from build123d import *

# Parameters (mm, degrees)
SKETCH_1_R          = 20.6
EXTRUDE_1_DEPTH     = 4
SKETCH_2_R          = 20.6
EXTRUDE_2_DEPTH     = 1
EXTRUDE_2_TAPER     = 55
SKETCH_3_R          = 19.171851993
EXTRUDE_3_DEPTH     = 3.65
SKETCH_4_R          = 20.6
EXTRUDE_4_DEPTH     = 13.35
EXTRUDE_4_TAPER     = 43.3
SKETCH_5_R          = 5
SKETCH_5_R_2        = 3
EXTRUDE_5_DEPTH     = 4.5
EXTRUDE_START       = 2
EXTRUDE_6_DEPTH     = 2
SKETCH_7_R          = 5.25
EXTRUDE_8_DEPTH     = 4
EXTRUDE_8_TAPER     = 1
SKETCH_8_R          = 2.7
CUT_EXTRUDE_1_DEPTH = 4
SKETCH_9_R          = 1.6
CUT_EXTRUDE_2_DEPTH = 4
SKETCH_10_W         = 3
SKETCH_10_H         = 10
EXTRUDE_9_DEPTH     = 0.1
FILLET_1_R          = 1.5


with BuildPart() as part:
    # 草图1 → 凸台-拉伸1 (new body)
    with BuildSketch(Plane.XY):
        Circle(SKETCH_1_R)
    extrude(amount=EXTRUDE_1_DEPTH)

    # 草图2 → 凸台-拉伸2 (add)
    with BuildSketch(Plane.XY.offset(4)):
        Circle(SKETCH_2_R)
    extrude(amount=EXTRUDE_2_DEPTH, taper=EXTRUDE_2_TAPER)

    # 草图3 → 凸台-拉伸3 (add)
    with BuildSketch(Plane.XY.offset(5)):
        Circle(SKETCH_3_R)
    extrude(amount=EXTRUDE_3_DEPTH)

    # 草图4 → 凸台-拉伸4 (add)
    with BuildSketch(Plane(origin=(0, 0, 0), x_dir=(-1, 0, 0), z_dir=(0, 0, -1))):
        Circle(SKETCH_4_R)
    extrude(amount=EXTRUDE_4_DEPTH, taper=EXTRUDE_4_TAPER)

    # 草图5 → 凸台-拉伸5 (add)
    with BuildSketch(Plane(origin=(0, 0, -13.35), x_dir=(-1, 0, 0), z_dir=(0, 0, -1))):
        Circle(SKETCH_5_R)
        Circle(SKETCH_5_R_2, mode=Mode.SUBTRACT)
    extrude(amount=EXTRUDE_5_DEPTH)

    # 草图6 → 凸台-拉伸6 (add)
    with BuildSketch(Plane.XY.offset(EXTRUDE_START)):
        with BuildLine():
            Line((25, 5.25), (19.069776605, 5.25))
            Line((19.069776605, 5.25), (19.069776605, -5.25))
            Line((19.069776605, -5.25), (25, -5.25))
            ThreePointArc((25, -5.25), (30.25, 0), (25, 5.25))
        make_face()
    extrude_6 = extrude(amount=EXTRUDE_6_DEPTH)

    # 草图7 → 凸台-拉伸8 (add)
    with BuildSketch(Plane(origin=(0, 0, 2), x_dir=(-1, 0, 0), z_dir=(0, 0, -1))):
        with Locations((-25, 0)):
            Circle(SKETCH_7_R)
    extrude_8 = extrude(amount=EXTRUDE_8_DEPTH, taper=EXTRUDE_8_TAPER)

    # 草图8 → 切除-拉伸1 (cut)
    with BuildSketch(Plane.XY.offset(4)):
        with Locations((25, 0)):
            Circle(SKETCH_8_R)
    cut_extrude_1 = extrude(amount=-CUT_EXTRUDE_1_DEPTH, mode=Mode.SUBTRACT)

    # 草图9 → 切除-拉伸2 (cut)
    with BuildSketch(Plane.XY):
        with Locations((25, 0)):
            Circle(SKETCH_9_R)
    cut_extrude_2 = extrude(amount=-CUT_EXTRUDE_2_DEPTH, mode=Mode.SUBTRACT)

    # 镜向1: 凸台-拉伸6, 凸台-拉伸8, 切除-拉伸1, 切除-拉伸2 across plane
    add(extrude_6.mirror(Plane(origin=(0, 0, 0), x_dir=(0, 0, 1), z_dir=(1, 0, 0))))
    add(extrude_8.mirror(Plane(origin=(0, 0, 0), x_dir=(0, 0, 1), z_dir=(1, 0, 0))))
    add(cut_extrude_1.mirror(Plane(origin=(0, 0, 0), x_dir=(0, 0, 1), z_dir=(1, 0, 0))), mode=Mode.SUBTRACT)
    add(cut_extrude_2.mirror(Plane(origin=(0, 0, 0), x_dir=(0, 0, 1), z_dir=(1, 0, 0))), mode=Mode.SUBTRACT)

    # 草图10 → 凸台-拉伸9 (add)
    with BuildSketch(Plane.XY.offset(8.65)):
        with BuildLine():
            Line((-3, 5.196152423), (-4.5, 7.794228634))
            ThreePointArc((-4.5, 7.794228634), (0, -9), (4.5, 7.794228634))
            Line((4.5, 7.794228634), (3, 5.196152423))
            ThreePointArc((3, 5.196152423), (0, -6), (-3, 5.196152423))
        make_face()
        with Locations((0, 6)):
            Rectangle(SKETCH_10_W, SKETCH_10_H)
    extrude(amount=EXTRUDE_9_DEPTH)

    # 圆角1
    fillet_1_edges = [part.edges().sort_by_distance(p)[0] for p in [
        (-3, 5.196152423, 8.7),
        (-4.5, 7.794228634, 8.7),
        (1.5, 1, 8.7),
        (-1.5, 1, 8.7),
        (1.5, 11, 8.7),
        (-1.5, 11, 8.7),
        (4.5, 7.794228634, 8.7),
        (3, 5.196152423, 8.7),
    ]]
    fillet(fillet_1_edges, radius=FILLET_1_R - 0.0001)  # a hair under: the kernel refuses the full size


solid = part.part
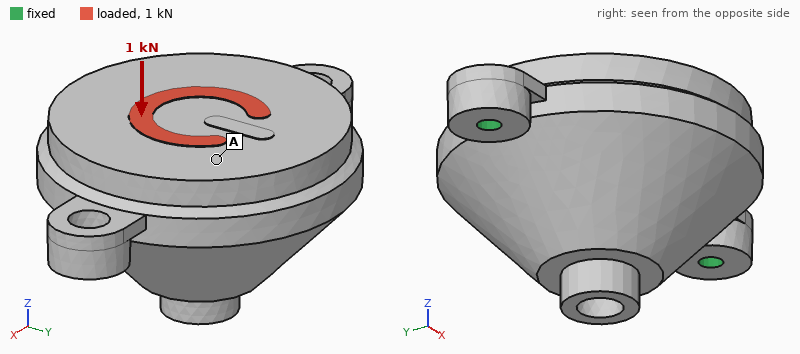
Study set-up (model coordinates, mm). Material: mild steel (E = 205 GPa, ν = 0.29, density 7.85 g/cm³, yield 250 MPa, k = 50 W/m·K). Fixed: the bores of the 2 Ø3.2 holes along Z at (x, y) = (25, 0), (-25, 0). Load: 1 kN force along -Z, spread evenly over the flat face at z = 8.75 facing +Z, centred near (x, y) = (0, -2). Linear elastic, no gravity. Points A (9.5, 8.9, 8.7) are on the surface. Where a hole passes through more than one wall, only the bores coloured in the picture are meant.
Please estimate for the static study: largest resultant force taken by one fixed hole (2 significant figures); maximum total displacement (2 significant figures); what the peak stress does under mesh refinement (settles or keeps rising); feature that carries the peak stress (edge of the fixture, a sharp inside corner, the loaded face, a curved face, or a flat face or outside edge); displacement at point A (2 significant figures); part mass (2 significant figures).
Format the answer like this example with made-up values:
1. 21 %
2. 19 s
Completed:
1. 610 N
2. 13 µm
3. keeps rising
4. edge of the fixture
5. 4.1 µm
6. 160 g
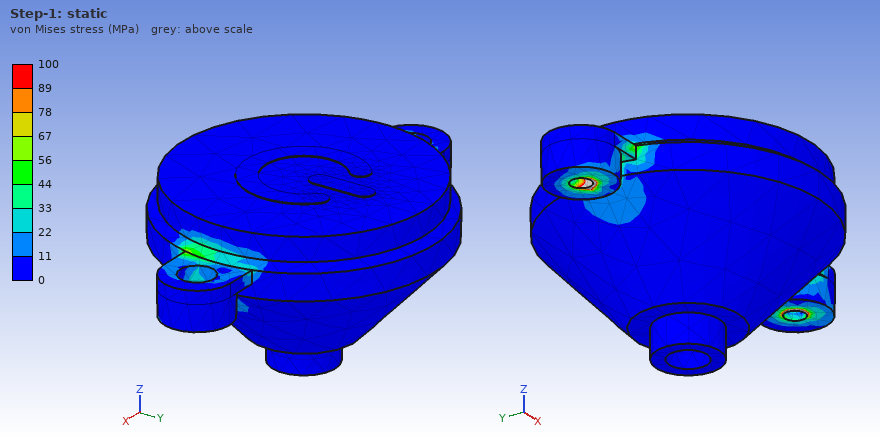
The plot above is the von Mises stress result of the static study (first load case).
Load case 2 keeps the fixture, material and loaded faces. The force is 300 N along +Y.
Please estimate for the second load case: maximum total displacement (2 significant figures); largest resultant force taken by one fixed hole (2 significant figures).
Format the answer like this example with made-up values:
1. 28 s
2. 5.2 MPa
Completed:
1. 17 µm
2. 150 N
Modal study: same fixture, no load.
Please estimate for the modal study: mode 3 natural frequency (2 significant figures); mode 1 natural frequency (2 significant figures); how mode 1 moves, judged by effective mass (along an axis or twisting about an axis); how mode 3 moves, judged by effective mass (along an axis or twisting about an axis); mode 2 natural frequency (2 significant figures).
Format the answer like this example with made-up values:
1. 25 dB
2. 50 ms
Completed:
1. 7600 Hz
2. 2200 Hz
3. twisting about X
4. along Y
5. 7300 Hz
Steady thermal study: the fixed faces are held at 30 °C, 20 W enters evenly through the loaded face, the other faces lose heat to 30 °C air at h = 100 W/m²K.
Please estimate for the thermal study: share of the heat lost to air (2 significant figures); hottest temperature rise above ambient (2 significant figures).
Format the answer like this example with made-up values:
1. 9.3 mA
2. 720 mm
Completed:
1. 53 %
2. 35 K
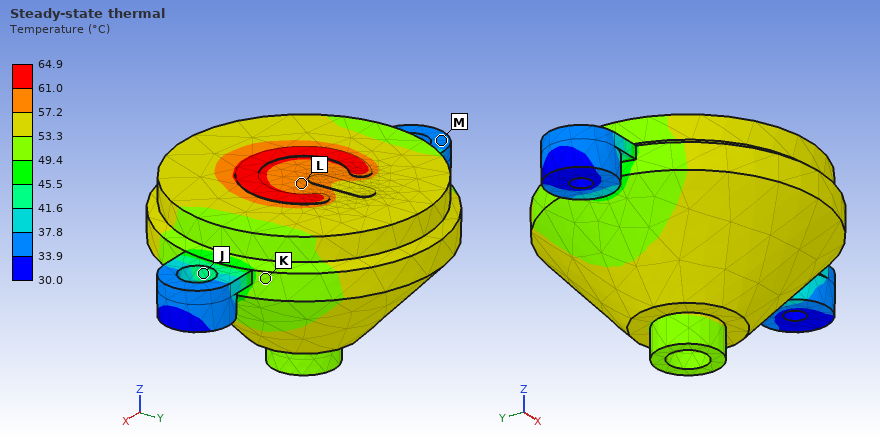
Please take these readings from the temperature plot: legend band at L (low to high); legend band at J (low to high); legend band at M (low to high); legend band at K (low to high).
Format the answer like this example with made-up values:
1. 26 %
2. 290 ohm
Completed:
1. 57.2 to 61.0 °C
2. 41.6 to 45.5 °C
3. 33.9 to 37.8 °C
4. 49.4 to 53.3 °C
